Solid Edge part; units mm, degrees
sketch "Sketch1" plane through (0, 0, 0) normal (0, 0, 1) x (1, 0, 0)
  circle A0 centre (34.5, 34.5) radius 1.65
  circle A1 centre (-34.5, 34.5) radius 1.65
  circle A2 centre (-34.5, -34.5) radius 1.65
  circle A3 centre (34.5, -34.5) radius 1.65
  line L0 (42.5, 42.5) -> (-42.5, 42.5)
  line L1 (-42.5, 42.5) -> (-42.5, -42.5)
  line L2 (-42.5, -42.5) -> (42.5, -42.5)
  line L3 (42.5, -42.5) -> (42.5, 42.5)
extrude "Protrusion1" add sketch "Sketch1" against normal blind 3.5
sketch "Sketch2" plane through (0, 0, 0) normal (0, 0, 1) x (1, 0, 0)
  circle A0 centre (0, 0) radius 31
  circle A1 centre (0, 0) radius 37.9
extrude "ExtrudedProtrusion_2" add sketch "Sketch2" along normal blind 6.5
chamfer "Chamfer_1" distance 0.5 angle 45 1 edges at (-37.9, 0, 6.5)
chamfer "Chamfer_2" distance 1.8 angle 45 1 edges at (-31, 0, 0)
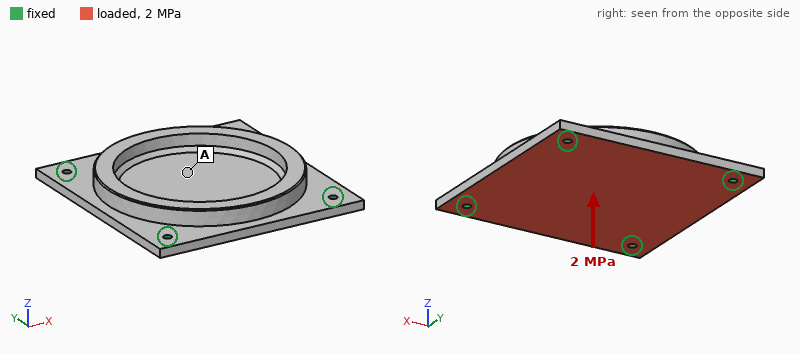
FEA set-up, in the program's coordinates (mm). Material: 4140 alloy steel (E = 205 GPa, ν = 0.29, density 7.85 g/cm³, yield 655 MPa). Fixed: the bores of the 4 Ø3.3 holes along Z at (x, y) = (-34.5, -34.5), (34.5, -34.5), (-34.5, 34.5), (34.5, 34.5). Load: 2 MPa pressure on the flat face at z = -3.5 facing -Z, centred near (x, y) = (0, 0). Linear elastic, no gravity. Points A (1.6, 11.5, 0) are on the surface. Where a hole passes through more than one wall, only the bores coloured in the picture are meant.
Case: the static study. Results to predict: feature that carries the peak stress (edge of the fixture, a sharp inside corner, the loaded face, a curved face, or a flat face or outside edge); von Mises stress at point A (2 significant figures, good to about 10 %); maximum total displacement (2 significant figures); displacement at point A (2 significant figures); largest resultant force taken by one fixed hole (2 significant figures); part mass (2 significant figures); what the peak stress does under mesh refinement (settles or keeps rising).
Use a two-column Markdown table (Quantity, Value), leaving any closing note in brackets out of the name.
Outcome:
| Quantity | Value |
|---|---|
| feature that carries the peak stress | edge of the fixture |
| von Mises stress at point A | 86 MPa |
| maximum total displacement | 0.17 mm |
| displacement at point A | 0.16 mm |
| largest resultant force taken by one fixed hole | 4.1 kN |
| part mass | 280 g |
| what the peak stress does under mesh refinement | keeps rising |
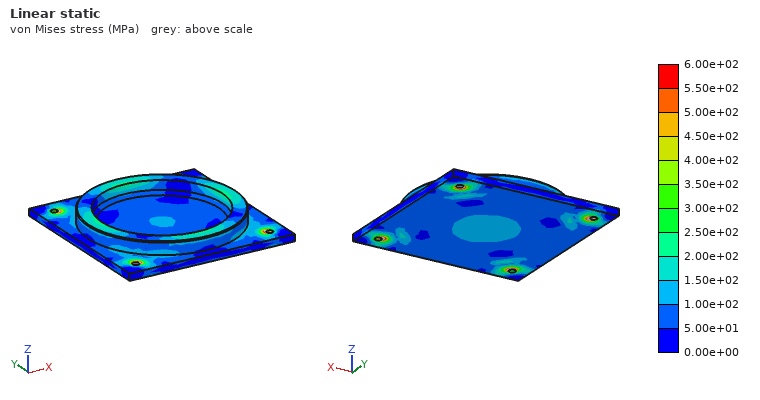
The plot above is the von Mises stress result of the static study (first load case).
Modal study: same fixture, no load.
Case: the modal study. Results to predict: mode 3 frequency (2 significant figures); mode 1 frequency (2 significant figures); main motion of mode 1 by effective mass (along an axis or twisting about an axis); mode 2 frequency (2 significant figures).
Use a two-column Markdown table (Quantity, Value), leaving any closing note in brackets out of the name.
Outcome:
| Quantity | Value |
|---|---|
| mode 3 frequency | 5200 Hz |
| mode 1 frequency | 3600 Hz |
| main motion of mode 1 by effective mass | along Z |
| mode 2 frequency | 5200 Hz |
